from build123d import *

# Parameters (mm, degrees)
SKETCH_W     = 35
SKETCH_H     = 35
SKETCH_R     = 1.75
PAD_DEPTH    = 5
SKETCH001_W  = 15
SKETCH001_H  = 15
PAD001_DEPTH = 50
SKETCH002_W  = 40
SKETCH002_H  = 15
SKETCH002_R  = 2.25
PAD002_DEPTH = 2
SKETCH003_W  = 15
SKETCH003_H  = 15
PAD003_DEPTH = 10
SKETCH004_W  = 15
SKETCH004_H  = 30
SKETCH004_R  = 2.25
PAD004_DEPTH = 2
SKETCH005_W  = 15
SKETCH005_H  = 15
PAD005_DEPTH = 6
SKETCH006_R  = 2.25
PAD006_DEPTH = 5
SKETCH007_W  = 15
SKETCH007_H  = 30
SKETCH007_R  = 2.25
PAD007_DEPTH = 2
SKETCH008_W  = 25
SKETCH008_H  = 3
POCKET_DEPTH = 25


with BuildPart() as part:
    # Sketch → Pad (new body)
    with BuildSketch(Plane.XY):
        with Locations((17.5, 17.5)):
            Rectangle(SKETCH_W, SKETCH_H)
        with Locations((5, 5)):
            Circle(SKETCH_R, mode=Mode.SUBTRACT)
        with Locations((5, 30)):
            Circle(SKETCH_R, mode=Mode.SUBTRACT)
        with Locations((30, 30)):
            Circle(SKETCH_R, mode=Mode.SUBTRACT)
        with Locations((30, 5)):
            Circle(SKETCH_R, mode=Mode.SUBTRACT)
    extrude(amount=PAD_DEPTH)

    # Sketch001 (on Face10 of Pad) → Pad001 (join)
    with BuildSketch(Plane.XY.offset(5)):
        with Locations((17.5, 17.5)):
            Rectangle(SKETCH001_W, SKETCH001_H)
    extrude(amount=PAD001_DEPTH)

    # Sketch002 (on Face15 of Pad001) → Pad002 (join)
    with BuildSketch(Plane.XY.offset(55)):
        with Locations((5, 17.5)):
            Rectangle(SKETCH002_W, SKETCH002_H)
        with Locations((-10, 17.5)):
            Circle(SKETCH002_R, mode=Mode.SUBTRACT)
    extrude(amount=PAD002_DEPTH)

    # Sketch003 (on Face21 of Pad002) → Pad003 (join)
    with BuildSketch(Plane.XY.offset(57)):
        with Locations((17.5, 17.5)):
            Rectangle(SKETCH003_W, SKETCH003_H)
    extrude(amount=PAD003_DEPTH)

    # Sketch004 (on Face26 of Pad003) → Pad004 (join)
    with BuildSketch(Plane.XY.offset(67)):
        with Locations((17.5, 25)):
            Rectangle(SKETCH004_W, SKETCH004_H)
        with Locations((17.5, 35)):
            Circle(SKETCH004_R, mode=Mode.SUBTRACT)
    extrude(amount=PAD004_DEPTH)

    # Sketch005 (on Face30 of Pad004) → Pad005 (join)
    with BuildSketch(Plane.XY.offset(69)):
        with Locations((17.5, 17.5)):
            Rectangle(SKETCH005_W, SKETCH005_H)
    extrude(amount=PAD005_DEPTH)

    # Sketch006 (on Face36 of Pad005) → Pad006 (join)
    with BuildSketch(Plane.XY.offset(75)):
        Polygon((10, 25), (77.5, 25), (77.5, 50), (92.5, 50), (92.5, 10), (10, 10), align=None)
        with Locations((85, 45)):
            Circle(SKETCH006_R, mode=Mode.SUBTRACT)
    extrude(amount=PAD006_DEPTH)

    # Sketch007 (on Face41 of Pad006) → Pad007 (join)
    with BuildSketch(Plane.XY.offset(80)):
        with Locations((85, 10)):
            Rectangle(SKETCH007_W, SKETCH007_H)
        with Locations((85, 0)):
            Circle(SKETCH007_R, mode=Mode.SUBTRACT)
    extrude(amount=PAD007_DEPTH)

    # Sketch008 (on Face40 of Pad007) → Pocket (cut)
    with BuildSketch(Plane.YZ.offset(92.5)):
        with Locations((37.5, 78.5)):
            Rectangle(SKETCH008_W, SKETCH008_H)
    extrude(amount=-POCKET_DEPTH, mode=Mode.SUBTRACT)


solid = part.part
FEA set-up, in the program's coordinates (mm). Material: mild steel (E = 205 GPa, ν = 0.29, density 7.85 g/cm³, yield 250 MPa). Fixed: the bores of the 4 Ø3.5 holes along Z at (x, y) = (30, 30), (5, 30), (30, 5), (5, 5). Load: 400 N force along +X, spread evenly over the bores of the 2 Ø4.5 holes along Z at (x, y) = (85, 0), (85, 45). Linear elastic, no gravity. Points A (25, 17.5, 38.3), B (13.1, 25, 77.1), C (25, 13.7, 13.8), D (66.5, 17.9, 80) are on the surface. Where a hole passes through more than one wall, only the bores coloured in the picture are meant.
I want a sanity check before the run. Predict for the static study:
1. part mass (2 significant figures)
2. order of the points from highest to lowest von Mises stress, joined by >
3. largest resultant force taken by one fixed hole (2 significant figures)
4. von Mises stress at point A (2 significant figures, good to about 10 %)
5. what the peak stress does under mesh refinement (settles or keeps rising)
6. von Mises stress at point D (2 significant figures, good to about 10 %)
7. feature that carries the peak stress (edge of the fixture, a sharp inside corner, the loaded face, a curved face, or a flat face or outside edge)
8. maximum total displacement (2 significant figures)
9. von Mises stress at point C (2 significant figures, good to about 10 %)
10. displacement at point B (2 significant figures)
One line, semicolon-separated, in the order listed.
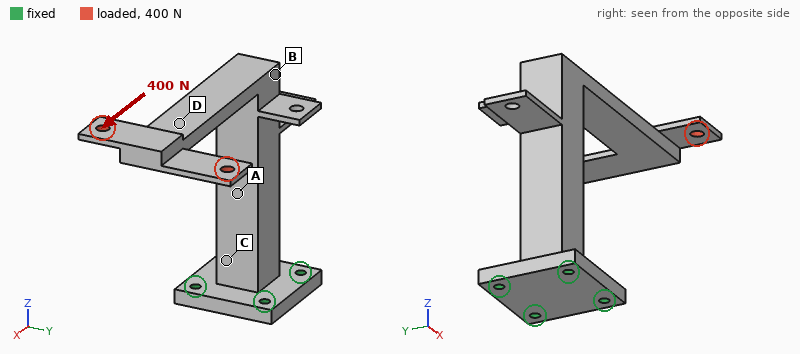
240 g; C > A > D > B; 710 N; 29 MPa; keeps rising; 13 MPa; edge of the fixture; 0.21 mm; 46 MPa; 0.096 mm
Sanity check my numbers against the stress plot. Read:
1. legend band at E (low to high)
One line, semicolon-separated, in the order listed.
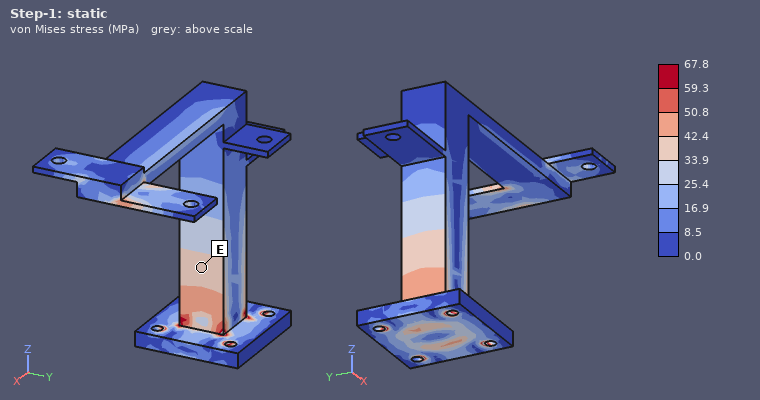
33.9 to 42.4 MPa
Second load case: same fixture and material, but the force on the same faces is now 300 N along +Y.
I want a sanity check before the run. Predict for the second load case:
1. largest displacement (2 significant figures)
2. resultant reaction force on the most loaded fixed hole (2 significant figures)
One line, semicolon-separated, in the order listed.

0.41 mm; 610 N
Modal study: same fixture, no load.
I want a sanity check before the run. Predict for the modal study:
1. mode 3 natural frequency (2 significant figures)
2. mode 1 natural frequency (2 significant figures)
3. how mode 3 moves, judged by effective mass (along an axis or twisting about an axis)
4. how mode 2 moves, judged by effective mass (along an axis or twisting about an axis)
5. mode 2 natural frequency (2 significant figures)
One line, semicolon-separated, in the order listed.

1100 Hz; 550 Hz; along X; along Y; 780 Hz
